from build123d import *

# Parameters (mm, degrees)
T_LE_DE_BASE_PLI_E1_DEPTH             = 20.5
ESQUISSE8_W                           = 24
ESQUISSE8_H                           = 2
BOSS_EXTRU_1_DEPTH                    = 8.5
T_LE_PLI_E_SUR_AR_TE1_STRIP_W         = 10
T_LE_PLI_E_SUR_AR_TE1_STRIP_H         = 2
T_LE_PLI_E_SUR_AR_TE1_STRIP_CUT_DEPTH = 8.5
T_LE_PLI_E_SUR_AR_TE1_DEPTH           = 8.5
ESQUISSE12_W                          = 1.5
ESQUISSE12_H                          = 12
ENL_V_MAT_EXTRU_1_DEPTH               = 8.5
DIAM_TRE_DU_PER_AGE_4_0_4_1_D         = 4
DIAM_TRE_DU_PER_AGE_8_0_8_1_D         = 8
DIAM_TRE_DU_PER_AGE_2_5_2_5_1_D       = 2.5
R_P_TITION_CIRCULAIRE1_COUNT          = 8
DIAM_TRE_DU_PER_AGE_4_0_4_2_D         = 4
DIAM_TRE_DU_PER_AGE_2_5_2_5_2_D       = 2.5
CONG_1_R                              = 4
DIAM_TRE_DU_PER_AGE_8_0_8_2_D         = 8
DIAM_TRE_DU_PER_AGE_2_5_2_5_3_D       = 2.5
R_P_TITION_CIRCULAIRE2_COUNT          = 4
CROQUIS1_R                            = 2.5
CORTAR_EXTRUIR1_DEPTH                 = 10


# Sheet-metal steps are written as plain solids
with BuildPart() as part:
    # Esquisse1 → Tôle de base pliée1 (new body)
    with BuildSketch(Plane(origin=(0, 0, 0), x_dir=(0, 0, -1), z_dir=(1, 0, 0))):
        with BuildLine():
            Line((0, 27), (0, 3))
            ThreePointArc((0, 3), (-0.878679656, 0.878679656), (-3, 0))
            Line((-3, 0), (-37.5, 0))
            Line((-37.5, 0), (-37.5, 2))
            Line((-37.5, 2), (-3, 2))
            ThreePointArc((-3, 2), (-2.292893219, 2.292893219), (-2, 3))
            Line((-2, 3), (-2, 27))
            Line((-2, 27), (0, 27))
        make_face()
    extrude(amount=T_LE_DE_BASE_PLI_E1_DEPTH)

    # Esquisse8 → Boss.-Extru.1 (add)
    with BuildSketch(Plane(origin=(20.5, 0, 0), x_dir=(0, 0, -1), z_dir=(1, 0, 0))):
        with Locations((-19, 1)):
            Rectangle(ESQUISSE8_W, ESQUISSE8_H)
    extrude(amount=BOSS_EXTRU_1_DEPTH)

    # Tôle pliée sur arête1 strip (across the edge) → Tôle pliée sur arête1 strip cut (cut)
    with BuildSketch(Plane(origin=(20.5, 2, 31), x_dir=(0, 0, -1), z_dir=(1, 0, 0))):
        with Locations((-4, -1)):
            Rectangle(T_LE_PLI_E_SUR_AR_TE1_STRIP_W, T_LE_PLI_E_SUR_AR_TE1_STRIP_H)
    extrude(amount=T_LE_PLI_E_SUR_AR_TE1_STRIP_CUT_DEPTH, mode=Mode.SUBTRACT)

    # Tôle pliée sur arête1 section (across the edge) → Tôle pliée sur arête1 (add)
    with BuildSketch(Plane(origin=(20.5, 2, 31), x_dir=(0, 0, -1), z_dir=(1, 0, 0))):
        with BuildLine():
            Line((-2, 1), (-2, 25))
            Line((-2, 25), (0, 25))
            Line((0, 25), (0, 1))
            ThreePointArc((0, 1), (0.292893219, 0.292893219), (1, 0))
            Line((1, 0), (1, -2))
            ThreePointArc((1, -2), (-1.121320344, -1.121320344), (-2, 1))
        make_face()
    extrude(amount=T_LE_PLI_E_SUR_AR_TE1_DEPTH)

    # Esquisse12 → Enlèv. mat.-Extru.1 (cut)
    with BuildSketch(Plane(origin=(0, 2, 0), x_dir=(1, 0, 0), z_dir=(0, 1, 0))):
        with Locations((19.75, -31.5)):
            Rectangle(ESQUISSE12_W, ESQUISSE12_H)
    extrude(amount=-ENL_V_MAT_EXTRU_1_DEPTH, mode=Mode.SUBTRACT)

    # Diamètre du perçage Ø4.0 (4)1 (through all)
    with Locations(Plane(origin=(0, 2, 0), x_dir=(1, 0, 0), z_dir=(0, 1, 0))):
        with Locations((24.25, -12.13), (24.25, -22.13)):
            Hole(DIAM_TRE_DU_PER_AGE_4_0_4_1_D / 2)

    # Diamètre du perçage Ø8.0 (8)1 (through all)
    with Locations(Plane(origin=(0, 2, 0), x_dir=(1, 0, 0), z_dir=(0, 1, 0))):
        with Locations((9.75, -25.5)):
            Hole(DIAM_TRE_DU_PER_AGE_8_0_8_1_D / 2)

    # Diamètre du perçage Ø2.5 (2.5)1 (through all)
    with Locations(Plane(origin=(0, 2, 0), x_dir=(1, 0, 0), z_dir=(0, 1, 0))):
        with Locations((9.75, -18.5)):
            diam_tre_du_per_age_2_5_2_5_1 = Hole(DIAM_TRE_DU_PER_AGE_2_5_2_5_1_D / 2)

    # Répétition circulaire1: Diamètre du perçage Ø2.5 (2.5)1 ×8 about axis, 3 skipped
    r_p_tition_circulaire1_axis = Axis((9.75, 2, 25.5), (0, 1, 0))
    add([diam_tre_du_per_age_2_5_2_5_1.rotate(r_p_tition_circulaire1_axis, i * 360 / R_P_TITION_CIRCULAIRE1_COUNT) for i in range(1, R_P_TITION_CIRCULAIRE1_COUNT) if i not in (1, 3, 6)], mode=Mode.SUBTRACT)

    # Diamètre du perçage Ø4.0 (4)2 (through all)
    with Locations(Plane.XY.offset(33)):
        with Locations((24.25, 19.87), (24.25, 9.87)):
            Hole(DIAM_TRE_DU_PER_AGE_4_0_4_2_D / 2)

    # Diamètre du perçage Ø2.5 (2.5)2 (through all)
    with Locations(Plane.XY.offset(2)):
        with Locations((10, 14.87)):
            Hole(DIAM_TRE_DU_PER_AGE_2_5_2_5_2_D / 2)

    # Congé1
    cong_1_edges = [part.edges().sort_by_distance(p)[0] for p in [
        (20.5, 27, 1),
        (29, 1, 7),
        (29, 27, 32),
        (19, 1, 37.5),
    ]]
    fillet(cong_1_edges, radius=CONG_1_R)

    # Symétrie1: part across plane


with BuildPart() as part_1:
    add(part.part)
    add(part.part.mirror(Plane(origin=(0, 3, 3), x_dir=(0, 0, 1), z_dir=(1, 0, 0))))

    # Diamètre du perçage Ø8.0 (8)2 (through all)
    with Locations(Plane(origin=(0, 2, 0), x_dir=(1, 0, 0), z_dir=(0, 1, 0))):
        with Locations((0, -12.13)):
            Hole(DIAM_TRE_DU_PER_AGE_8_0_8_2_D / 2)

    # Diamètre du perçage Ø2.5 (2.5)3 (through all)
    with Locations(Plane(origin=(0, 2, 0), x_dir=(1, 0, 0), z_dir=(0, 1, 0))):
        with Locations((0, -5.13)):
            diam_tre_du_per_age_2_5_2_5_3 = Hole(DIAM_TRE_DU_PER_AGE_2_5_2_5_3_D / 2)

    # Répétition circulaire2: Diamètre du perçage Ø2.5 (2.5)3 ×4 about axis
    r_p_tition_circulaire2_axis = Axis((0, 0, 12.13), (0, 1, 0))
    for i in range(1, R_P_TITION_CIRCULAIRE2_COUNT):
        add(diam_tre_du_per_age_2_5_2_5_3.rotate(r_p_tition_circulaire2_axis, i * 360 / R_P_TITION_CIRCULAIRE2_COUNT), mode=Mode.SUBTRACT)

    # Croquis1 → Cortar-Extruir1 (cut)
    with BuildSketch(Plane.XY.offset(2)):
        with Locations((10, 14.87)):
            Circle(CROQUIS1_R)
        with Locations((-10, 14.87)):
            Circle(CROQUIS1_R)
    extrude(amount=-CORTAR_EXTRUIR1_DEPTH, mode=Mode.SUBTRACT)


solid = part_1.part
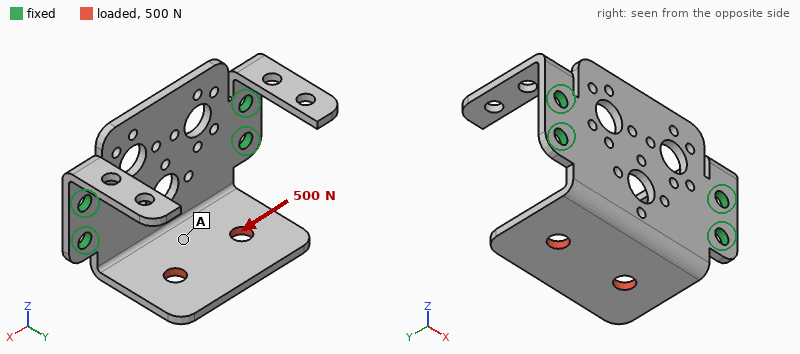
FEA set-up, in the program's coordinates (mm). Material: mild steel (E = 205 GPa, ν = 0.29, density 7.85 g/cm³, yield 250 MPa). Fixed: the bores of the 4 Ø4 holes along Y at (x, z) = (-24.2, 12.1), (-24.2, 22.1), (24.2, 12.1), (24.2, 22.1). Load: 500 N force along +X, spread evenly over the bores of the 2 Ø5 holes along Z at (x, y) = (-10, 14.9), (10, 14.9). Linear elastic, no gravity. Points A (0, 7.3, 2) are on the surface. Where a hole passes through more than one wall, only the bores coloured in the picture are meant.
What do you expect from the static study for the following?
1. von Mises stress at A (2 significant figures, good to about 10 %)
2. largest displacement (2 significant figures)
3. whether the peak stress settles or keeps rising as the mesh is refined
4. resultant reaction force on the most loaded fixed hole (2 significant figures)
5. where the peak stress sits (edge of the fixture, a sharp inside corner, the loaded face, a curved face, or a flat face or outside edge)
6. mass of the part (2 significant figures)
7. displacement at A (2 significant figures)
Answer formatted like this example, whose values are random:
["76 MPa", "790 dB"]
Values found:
["40 MPa", "75 µm", "keeps rising", "310 N", "edge of the fixture", "46 g", "15 µm"]
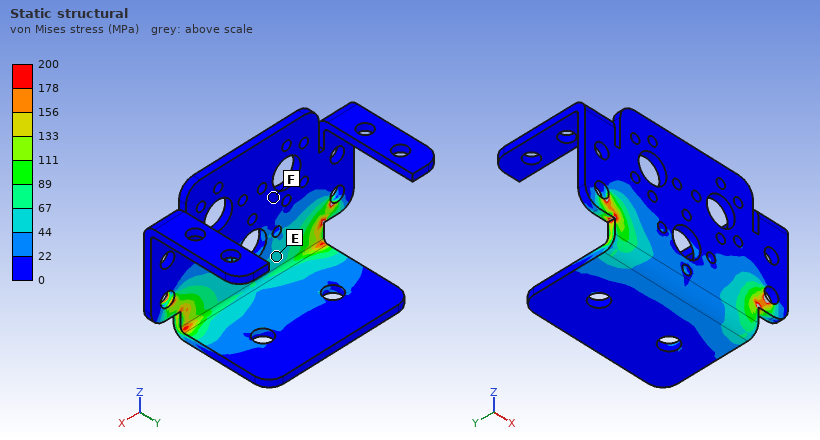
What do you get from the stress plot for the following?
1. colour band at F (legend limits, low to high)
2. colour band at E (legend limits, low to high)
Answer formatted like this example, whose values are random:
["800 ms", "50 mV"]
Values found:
["0 to 22 MPa", "44 to 67 MPa"]
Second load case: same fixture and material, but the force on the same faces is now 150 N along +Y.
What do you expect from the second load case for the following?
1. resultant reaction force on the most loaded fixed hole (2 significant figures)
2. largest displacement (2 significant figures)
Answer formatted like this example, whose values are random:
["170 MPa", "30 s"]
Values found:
["110 N", "70 µm"]
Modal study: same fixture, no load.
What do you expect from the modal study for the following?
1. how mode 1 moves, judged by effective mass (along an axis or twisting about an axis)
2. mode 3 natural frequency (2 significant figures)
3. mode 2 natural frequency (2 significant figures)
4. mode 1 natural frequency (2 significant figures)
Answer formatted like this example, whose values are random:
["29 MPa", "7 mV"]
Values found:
["along Z", "1700 Hz", "1700 Hz", "1300 Hz"]
